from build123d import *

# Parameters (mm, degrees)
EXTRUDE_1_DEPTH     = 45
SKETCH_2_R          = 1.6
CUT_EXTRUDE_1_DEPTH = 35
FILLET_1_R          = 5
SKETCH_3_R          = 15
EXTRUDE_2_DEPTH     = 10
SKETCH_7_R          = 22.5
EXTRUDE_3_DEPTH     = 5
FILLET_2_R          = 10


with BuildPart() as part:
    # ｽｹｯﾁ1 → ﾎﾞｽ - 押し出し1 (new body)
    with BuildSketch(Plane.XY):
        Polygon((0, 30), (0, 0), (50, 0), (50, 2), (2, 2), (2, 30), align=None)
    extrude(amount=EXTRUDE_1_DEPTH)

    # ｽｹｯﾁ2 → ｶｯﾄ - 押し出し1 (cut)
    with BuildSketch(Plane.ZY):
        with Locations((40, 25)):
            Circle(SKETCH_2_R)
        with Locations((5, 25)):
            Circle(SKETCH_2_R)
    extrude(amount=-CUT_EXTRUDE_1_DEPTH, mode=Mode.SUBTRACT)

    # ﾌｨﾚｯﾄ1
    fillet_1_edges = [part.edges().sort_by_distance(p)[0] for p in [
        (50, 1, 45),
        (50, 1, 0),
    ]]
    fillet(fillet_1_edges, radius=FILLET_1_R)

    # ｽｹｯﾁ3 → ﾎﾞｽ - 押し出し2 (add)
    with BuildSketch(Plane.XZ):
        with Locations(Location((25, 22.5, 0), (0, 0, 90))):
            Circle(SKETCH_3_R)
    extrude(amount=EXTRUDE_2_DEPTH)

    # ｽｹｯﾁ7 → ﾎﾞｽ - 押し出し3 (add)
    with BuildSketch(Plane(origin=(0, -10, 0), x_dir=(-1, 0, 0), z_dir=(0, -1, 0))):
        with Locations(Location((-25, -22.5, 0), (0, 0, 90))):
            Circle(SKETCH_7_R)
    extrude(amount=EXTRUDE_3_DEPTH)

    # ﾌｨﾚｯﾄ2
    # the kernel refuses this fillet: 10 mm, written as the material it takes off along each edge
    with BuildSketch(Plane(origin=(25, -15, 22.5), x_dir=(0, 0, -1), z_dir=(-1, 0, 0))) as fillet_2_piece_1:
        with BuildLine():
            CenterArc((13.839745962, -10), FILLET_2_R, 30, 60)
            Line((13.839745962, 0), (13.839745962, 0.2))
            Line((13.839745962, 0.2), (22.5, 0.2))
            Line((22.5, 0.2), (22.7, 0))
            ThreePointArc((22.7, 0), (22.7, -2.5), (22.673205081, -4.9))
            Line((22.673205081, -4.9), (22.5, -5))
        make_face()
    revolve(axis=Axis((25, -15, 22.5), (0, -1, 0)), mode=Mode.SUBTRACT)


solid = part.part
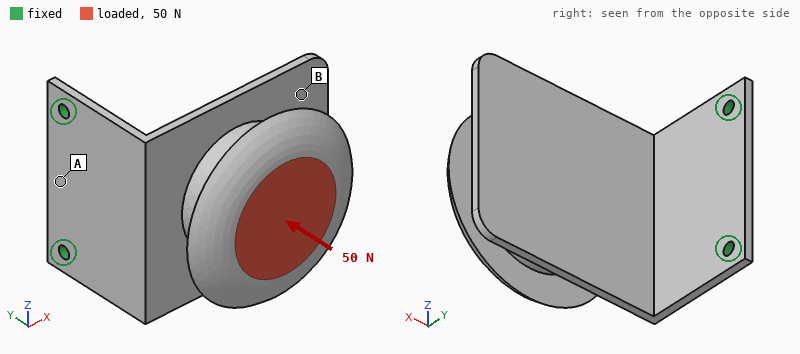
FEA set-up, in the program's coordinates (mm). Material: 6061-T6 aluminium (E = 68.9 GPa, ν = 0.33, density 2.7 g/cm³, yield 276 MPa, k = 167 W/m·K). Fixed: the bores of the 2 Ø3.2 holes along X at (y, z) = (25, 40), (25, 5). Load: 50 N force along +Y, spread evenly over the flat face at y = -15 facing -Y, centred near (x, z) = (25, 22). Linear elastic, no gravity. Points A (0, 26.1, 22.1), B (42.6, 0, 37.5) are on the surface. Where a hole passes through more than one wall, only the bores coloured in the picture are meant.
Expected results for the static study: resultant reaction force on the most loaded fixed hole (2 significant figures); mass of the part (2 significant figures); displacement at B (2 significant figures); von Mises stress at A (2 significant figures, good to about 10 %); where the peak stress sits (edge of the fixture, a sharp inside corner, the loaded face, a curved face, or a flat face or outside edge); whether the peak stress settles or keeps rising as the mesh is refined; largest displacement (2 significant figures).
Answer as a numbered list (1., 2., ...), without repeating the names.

1. 27 N
2. 55 g
3. 0.78 mm
4. 10 MPa
5. edge of the fixture
6. keeps rising
7. 0.93 mm
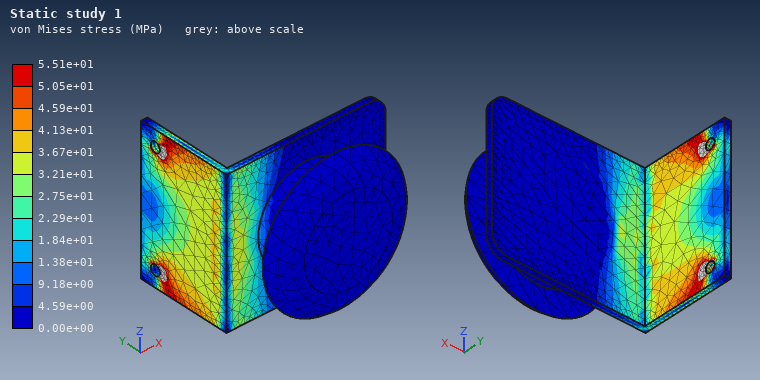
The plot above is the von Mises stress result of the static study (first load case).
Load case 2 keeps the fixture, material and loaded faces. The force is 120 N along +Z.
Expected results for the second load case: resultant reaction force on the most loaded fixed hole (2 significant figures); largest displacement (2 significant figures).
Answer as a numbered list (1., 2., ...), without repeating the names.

1. 170 N
2. 0.38 mm
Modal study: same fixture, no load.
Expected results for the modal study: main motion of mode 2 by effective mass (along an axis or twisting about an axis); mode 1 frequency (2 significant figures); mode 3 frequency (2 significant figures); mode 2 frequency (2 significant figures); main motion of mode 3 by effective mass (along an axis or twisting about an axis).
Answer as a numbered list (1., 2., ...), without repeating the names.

1. along Z
2. 180 Hz
3. 870 Hz
4. 490 Hz
5. along X
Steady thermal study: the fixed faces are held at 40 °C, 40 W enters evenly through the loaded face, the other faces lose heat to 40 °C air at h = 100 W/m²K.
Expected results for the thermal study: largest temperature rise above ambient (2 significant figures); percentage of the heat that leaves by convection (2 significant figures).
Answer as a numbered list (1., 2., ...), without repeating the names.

1. 44 K
2. 73 %
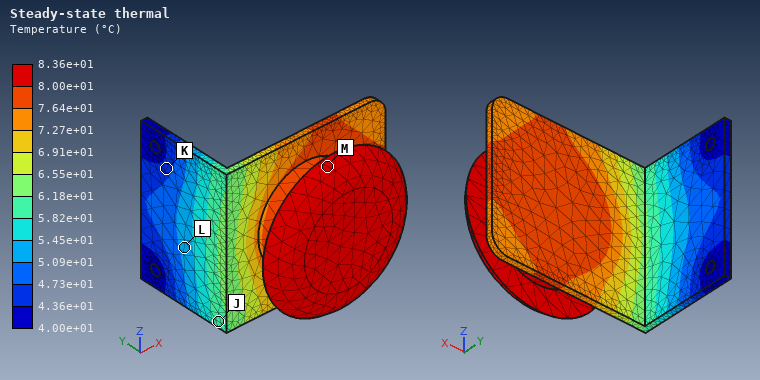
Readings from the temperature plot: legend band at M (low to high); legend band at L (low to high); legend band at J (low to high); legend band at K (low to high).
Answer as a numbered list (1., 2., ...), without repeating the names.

1. 8.00e+01 to 8.36e+01 °C
2. 5.09e+01 to 5.45e+01 °C
3. 5.82e+01 to 6.18e+01 °C
4. 4.36e+01 to 4.73e+01 °C
